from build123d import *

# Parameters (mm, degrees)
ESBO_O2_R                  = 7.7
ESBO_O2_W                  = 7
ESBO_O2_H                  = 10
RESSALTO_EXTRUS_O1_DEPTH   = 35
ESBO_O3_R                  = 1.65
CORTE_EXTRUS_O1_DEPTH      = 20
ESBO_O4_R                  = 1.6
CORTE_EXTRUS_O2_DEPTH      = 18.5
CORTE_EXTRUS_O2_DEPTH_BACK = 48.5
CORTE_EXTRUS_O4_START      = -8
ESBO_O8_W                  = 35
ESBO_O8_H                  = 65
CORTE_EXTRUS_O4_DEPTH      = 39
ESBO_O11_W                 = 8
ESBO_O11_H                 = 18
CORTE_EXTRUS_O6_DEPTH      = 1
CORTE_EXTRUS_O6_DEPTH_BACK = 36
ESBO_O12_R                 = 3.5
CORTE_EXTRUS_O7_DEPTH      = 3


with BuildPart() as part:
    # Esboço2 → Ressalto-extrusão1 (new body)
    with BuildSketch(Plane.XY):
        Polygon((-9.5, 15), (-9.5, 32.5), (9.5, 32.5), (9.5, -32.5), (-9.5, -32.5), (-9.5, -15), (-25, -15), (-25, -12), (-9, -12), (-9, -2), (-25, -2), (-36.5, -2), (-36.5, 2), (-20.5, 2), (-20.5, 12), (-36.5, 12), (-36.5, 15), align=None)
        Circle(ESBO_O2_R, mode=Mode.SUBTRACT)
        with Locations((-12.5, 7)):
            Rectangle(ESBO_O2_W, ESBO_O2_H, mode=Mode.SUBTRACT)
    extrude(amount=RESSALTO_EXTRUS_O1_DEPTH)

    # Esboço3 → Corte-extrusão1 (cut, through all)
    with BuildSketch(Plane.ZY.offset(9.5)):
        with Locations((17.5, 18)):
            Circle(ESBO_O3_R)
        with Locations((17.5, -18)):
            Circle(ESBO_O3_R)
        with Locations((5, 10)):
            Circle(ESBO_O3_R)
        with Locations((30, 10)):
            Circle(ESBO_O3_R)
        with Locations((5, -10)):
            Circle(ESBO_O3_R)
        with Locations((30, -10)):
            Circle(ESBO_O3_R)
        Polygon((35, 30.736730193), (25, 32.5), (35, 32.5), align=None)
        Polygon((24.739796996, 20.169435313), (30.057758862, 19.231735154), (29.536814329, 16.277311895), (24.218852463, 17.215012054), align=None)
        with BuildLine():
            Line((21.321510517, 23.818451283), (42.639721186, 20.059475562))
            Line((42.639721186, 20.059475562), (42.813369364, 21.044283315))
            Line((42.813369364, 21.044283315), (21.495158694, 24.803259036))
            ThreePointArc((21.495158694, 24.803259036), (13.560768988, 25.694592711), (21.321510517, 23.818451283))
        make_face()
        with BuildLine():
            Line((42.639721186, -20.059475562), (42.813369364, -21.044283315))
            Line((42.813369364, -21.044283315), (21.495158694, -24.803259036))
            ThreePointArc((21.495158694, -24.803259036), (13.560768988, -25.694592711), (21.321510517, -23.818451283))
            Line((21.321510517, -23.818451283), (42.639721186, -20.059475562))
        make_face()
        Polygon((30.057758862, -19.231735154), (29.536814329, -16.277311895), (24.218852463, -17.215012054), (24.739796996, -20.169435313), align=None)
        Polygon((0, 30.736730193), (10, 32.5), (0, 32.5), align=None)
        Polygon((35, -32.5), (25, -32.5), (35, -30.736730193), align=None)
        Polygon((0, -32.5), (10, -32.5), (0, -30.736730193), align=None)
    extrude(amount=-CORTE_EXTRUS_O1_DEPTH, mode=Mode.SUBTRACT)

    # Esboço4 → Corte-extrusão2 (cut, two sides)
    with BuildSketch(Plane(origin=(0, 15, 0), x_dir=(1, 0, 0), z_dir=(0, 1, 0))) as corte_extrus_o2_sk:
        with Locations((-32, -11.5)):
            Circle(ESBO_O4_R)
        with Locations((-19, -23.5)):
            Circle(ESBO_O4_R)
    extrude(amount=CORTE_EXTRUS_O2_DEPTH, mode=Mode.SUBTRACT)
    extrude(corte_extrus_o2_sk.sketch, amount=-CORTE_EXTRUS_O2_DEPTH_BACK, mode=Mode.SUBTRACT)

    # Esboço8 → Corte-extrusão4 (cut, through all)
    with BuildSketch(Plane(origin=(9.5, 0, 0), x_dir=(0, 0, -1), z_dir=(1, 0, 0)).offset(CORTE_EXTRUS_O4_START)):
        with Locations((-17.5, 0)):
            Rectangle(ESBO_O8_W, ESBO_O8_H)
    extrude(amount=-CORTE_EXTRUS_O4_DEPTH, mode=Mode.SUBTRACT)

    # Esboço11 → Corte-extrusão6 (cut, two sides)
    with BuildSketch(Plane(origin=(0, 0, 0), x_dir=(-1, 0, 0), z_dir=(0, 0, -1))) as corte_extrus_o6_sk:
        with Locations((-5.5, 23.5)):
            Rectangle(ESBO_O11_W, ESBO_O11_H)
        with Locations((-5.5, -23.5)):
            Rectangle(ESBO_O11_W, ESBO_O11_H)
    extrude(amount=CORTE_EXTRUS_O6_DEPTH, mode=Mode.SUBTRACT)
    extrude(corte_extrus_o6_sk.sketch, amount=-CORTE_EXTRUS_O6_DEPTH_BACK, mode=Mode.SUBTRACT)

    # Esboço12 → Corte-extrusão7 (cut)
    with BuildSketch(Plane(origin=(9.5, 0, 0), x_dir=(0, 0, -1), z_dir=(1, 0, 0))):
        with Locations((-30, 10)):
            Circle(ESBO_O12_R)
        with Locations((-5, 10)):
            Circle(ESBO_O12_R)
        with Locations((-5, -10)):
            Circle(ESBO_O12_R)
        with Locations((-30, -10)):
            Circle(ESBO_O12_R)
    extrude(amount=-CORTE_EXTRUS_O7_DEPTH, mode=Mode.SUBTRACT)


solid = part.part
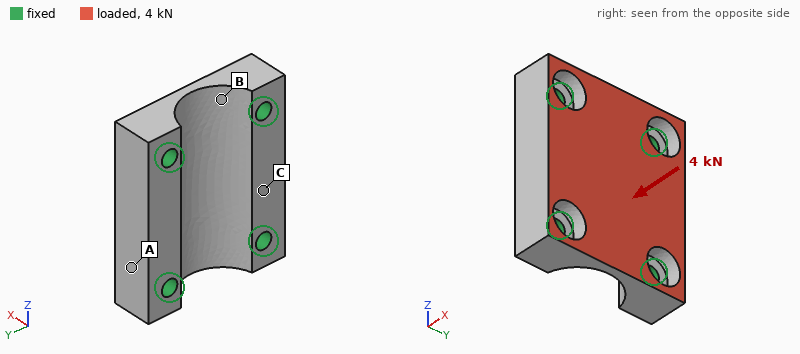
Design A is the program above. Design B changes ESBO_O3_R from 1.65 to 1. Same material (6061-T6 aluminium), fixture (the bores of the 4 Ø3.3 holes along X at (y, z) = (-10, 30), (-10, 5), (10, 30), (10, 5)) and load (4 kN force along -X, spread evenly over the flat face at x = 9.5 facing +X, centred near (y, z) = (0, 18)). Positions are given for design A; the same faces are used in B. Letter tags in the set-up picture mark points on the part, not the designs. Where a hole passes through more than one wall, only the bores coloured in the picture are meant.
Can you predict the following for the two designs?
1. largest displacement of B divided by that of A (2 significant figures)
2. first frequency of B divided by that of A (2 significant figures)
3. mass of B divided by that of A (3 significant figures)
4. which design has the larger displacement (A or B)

1.2
0.89
1.02
B
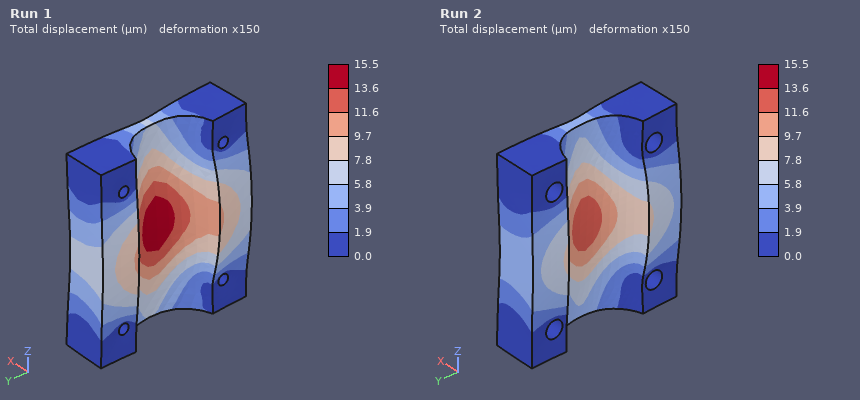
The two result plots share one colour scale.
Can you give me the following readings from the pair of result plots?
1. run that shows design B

Run 1
